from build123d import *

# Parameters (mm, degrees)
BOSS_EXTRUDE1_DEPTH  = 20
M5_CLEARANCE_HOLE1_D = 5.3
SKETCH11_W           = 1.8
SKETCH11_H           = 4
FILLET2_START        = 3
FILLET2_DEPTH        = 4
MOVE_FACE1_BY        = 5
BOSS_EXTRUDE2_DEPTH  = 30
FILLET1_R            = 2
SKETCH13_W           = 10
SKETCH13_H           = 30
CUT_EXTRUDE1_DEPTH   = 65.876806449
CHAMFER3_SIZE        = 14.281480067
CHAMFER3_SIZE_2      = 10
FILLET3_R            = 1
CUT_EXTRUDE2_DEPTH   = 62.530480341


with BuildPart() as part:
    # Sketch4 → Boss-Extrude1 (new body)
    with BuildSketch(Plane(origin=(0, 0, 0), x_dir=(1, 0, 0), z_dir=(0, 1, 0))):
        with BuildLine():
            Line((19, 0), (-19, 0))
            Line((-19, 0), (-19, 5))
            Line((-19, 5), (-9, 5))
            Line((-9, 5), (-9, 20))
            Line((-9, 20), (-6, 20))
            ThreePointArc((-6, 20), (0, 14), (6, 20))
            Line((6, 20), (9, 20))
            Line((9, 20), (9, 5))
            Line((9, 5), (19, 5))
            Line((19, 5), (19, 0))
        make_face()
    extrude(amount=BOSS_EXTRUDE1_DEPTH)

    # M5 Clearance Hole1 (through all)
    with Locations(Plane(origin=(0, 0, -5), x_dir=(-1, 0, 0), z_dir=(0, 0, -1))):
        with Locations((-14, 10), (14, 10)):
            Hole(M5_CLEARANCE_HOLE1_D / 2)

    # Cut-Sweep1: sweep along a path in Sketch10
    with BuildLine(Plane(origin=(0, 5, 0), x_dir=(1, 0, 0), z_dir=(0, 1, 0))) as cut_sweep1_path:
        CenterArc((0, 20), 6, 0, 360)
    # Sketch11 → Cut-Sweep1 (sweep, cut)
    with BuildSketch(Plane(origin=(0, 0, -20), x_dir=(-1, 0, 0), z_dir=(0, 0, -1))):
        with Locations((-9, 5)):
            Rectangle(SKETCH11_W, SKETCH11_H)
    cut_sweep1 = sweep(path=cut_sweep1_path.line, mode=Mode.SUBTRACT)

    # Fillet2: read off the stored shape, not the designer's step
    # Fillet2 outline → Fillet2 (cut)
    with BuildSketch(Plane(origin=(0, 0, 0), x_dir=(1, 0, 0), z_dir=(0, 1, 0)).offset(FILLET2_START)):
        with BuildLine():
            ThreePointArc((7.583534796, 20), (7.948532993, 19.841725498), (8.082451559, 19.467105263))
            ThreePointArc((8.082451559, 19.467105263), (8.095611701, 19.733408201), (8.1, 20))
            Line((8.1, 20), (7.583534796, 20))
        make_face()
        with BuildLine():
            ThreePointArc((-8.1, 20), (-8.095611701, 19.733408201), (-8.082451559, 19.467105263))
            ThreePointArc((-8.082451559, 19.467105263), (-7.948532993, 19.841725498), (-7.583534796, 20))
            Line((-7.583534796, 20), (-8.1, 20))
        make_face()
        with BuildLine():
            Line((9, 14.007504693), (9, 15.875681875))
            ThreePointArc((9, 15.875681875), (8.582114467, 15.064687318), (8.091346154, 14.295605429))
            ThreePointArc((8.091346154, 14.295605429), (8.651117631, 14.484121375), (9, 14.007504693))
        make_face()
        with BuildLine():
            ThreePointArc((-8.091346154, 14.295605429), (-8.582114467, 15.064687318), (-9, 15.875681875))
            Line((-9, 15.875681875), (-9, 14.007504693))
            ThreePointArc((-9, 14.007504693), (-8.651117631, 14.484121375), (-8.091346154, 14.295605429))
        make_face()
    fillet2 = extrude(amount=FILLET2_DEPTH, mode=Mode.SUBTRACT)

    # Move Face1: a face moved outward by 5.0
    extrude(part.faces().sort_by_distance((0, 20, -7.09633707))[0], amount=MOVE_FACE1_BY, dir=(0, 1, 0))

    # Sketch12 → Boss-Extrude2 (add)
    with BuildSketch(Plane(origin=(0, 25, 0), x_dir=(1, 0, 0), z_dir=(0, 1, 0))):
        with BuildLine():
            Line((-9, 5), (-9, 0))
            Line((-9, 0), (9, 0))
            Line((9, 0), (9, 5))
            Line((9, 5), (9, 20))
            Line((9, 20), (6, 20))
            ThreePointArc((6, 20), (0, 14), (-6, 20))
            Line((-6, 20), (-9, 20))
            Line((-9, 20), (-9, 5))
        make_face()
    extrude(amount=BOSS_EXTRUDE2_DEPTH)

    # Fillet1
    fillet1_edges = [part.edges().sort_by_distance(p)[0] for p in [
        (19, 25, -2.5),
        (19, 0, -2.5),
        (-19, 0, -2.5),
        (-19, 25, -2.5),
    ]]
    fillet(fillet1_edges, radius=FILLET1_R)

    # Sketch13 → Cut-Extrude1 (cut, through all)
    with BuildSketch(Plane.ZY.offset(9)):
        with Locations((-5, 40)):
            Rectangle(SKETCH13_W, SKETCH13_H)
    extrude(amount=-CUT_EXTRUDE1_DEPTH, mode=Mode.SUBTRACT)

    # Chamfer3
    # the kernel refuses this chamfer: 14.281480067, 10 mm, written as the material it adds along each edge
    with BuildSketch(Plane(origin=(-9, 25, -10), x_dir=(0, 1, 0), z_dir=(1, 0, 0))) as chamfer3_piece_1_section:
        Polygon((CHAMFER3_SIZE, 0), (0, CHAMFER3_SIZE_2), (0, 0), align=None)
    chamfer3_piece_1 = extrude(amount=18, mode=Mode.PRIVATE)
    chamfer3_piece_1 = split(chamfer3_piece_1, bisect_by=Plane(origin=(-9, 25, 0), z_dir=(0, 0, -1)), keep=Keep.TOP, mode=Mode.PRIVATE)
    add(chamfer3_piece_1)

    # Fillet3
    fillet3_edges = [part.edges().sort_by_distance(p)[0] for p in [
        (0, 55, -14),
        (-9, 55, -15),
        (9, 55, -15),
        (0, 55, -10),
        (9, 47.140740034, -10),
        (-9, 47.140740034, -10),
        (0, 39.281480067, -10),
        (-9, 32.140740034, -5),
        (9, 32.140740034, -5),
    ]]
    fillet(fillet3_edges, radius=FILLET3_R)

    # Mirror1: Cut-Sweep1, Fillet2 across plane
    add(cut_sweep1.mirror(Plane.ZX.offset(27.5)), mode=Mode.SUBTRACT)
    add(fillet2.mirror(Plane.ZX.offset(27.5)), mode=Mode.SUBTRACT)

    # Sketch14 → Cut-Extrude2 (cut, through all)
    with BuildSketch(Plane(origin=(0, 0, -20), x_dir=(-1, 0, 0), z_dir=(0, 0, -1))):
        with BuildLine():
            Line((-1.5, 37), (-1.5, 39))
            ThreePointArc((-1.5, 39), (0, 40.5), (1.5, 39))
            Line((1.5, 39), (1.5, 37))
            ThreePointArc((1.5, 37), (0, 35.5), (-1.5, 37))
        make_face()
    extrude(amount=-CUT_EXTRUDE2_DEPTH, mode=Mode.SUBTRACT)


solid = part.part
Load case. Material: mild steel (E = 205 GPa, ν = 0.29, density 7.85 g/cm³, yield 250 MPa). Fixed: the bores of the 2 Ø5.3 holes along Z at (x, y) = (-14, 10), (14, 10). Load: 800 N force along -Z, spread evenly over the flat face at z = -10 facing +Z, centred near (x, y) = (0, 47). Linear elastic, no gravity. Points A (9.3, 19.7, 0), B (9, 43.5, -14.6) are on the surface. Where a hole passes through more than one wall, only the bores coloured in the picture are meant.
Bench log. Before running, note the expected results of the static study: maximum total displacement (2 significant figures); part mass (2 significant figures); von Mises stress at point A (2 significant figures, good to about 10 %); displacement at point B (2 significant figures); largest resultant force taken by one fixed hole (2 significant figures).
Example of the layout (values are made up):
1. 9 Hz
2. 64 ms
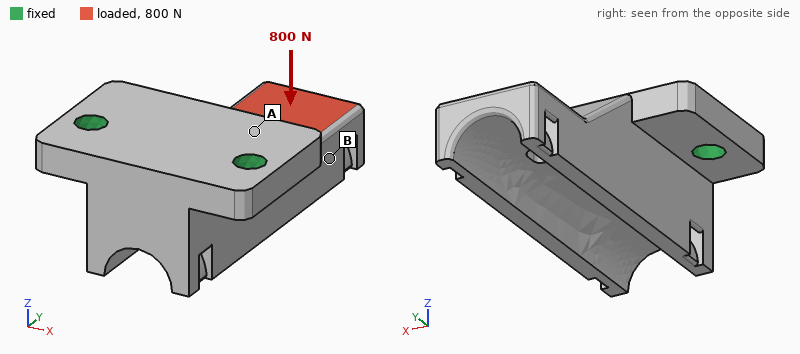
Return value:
1. 72 µm
2. 110 g
3. 40 MPa
4. 48 µm
5. 480 N
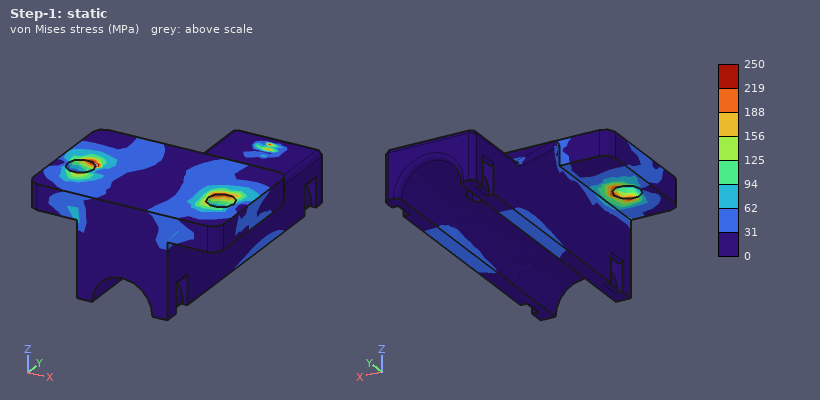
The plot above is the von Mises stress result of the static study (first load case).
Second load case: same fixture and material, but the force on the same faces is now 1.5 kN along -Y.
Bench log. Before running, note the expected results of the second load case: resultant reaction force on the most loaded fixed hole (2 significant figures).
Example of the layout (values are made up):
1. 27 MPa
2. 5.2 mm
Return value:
1. 760 N
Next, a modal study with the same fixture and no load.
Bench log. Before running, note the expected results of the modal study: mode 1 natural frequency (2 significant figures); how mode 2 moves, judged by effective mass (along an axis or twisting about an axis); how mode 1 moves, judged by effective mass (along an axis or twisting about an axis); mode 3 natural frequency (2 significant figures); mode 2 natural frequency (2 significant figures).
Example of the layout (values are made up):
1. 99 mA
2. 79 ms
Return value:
1. 3800 Hz
2. along X
3. along Z
4. 16 kHz
5. 9300 Hz
